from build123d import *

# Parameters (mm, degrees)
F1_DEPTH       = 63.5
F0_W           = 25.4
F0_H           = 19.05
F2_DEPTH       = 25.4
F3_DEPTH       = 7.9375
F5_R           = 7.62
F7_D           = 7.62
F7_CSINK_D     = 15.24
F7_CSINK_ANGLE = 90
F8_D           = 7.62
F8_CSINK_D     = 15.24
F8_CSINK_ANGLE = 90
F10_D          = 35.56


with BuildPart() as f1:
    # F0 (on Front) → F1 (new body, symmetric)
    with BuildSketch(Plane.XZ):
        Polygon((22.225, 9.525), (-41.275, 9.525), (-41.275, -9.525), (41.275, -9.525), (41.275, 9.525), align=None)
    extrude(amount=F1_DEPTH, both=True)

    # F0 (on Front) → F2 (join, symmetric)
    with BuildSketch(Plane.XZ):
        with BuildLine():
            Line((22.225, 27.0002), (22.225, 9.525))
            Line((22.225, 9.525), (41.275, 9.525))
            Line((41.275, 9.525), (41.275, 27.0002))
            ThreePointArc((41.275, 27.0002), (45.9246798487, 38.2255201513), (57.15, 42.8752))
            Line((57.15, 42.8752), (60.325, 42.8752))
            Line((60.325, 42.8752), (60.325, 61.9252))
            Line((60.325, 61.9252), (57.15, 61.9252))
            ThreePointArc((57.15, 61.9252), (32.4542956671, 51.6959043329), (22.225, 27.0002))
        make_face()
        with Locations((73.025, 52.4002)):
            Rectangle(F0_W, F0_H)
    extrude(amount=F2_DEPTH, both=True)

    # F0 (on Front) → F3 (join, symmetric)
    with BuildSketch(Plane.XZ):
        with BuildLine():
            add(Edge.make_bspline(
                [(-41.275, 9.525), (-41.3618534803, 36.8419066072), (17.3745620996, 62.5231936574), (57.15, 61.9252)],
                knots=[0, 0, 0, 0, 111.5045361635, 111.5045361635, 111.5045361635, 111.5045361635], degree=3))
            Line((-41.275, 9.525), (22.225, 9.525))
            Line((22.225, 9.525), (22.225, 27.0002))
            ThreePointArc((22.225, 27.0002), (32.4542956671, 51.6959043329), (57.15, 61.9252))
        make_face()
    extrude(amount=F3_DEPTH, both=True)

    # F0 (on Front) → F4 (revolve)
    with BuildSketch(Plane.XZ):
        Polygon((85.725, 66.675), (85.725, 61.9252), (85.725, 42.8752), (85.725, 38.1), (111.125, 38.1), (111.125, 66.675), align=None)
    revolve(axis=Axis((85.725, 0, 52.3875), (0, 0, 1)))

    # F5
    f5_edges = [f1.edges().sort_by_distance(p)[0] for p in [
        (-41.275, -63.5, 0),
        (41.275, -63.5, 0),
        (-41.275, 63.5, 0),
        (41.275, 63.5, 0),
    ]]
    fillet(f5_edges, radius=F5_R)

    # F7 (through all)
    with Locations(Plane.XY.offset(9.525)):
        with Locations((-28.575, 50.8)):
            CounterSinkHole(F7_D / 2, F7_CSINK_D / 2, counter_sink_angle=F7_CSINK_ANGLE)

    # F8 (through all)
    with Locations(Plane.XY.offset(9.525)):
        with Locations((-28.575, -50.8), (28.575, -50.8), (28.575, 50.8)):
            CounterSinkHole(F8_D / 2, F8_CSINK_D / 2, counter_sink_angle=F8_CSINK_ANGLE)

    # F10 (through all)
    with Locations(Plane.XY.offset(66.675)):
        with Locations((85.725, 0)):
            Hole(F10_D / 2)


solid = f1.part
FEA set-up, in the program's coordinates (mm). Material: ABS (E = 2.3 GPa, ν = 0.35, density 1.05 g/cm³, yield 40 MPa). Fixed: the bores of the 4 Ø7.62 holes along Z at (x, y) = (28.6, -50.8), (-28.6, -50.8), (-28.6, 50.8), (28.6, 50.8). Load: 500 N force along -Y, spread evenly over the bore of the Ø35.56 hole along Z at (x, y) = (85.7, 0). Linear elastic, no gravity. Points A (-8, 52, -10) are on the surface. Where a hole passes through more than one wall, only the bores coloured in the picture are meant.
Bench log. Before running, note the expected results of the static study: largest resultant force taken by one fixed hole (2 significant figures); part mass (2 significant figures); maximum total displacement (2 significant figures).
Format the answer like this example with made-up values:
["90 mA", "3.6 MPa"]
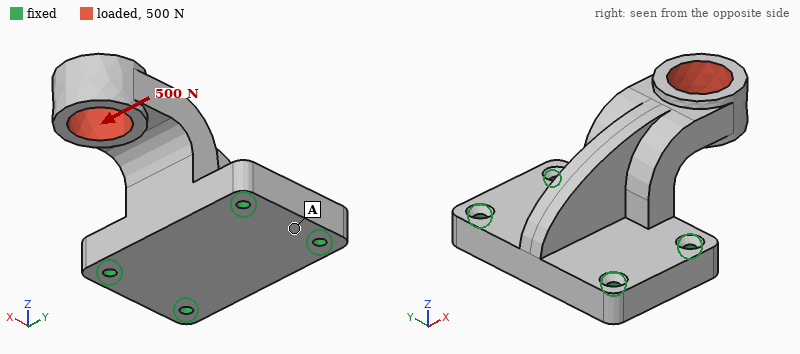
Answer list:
["420 N", "340 g", "0.94 mm"]
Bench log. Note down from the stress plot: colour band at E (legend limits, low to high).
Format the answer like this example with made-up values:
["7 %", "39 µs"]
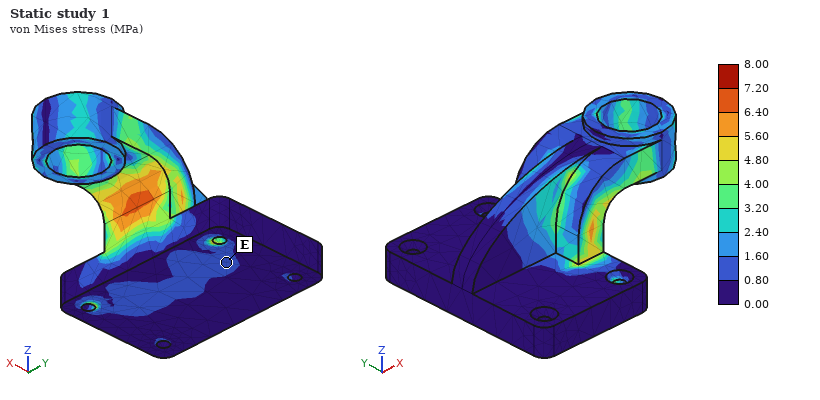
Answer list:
["0.80 to 1.60 MPa"]
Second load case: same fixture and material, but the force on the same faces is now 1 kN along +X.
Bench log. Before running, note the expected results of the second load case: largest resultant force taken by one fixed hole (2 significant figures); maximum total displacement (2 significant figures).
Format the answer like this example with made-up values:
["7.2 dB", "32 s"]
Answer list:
["580 N", "0.77 mm"]
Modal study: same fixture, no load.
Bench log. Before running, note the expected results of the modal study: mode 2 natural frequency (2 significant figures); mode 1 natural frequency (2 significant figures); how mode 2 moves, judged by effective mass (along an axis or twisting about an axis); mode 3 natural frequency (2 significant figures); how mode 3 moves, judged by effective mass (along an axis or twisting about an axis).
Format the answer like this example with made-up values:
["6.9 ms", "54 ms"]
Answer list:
["670 Hz", "580 Hz", "along Y", "1200 Hz", "along X"]
